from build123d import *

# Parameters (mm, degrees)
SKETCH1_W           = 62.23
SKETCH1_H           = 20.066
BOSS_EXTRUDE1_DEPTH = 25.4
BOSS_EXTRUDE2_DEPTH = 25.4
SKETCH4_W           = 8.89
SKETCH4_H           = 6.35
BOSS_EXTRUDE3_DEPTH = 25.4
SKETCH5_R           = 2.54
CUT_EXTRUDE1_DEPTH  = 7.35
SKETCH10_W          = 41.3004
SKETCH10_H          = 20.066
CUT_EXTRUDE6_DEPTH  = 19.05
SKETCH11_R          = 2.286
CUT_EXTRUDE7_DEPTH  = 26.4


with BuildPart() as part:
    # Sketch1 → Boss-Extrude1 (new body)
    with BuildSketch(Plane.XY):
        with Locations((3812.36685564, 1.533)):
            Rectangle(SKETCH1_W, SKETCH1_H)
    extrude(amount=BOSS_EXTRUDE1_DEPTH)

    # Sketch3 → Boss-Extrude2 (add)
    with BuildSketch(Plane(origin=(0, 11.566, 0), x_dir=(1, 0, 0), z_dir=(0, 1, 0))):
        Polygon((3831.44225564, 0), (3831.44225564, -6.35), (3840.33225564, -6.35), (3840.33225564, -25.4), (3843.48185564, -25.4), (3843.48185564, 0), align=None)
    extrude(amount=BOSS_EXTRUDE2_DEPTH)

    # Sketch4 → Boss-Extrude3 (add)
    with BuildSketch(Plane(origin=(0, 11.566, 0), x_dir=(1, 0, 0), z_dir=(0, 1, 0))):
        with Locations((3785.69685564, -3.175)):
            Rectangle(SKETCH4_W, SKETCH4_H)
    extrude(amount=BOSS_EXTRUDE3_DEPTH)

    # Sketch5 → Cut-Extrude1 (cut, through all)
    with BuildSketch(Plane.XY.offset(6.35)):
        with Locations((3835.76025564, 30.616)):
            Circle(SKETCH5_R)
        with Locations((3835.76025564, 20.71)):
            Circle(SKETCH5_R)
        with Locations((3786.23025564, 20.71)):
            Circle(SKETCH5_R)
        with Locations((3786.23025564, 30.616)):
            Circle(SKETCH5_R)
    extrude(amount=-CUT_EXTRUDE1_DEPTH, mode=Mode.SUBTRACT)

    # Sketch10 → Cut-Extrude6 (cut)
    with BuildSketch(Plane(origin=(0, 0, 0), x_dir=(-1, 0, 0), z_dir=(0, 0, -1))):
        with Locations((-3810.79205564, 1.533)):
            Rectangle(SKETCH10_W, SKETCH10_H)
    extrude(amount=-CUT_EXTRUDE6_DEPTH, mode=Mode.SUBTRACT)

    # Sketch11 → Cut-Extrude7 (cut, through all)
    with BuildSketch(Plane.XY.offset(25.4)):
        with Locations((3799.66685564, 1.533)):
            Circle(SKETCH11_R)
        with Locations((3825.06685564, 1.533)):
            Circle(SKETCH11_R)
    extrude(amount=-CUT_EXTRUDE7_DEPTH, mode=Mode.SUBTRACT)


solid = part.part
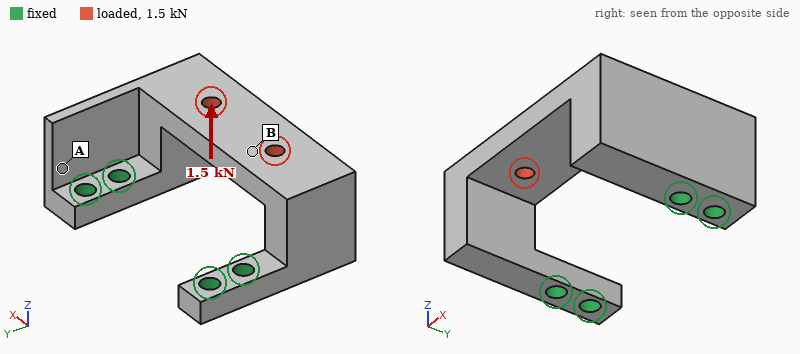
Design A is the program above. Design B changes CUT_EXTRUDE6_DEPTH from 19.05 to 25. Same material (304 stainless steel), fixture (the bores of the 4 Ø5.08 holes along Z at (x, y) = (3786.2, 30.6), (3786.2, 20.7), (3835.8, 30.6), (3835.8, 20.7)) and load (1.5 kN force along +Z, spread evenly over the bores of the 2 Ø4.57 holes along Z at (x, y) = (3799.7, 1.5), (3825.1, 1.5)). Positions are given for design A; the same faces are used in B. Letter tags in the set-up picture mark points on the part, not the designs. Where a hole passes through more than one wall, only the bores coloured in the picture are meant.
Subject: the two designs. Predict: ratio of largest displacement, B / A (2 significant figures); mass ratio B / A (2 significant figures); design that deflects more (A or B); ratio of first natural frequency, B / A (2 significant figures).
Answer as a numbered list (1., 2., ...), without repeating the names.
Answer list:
1. 140
2. 0.76
3. B
4. 0.49
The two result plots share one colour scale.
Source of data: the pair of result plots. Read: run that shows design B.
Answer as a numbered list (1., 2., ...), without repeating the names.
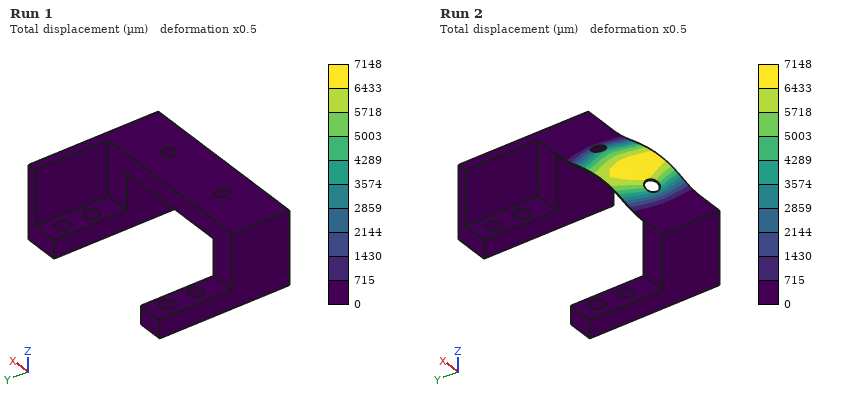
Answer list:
1. Run 2
